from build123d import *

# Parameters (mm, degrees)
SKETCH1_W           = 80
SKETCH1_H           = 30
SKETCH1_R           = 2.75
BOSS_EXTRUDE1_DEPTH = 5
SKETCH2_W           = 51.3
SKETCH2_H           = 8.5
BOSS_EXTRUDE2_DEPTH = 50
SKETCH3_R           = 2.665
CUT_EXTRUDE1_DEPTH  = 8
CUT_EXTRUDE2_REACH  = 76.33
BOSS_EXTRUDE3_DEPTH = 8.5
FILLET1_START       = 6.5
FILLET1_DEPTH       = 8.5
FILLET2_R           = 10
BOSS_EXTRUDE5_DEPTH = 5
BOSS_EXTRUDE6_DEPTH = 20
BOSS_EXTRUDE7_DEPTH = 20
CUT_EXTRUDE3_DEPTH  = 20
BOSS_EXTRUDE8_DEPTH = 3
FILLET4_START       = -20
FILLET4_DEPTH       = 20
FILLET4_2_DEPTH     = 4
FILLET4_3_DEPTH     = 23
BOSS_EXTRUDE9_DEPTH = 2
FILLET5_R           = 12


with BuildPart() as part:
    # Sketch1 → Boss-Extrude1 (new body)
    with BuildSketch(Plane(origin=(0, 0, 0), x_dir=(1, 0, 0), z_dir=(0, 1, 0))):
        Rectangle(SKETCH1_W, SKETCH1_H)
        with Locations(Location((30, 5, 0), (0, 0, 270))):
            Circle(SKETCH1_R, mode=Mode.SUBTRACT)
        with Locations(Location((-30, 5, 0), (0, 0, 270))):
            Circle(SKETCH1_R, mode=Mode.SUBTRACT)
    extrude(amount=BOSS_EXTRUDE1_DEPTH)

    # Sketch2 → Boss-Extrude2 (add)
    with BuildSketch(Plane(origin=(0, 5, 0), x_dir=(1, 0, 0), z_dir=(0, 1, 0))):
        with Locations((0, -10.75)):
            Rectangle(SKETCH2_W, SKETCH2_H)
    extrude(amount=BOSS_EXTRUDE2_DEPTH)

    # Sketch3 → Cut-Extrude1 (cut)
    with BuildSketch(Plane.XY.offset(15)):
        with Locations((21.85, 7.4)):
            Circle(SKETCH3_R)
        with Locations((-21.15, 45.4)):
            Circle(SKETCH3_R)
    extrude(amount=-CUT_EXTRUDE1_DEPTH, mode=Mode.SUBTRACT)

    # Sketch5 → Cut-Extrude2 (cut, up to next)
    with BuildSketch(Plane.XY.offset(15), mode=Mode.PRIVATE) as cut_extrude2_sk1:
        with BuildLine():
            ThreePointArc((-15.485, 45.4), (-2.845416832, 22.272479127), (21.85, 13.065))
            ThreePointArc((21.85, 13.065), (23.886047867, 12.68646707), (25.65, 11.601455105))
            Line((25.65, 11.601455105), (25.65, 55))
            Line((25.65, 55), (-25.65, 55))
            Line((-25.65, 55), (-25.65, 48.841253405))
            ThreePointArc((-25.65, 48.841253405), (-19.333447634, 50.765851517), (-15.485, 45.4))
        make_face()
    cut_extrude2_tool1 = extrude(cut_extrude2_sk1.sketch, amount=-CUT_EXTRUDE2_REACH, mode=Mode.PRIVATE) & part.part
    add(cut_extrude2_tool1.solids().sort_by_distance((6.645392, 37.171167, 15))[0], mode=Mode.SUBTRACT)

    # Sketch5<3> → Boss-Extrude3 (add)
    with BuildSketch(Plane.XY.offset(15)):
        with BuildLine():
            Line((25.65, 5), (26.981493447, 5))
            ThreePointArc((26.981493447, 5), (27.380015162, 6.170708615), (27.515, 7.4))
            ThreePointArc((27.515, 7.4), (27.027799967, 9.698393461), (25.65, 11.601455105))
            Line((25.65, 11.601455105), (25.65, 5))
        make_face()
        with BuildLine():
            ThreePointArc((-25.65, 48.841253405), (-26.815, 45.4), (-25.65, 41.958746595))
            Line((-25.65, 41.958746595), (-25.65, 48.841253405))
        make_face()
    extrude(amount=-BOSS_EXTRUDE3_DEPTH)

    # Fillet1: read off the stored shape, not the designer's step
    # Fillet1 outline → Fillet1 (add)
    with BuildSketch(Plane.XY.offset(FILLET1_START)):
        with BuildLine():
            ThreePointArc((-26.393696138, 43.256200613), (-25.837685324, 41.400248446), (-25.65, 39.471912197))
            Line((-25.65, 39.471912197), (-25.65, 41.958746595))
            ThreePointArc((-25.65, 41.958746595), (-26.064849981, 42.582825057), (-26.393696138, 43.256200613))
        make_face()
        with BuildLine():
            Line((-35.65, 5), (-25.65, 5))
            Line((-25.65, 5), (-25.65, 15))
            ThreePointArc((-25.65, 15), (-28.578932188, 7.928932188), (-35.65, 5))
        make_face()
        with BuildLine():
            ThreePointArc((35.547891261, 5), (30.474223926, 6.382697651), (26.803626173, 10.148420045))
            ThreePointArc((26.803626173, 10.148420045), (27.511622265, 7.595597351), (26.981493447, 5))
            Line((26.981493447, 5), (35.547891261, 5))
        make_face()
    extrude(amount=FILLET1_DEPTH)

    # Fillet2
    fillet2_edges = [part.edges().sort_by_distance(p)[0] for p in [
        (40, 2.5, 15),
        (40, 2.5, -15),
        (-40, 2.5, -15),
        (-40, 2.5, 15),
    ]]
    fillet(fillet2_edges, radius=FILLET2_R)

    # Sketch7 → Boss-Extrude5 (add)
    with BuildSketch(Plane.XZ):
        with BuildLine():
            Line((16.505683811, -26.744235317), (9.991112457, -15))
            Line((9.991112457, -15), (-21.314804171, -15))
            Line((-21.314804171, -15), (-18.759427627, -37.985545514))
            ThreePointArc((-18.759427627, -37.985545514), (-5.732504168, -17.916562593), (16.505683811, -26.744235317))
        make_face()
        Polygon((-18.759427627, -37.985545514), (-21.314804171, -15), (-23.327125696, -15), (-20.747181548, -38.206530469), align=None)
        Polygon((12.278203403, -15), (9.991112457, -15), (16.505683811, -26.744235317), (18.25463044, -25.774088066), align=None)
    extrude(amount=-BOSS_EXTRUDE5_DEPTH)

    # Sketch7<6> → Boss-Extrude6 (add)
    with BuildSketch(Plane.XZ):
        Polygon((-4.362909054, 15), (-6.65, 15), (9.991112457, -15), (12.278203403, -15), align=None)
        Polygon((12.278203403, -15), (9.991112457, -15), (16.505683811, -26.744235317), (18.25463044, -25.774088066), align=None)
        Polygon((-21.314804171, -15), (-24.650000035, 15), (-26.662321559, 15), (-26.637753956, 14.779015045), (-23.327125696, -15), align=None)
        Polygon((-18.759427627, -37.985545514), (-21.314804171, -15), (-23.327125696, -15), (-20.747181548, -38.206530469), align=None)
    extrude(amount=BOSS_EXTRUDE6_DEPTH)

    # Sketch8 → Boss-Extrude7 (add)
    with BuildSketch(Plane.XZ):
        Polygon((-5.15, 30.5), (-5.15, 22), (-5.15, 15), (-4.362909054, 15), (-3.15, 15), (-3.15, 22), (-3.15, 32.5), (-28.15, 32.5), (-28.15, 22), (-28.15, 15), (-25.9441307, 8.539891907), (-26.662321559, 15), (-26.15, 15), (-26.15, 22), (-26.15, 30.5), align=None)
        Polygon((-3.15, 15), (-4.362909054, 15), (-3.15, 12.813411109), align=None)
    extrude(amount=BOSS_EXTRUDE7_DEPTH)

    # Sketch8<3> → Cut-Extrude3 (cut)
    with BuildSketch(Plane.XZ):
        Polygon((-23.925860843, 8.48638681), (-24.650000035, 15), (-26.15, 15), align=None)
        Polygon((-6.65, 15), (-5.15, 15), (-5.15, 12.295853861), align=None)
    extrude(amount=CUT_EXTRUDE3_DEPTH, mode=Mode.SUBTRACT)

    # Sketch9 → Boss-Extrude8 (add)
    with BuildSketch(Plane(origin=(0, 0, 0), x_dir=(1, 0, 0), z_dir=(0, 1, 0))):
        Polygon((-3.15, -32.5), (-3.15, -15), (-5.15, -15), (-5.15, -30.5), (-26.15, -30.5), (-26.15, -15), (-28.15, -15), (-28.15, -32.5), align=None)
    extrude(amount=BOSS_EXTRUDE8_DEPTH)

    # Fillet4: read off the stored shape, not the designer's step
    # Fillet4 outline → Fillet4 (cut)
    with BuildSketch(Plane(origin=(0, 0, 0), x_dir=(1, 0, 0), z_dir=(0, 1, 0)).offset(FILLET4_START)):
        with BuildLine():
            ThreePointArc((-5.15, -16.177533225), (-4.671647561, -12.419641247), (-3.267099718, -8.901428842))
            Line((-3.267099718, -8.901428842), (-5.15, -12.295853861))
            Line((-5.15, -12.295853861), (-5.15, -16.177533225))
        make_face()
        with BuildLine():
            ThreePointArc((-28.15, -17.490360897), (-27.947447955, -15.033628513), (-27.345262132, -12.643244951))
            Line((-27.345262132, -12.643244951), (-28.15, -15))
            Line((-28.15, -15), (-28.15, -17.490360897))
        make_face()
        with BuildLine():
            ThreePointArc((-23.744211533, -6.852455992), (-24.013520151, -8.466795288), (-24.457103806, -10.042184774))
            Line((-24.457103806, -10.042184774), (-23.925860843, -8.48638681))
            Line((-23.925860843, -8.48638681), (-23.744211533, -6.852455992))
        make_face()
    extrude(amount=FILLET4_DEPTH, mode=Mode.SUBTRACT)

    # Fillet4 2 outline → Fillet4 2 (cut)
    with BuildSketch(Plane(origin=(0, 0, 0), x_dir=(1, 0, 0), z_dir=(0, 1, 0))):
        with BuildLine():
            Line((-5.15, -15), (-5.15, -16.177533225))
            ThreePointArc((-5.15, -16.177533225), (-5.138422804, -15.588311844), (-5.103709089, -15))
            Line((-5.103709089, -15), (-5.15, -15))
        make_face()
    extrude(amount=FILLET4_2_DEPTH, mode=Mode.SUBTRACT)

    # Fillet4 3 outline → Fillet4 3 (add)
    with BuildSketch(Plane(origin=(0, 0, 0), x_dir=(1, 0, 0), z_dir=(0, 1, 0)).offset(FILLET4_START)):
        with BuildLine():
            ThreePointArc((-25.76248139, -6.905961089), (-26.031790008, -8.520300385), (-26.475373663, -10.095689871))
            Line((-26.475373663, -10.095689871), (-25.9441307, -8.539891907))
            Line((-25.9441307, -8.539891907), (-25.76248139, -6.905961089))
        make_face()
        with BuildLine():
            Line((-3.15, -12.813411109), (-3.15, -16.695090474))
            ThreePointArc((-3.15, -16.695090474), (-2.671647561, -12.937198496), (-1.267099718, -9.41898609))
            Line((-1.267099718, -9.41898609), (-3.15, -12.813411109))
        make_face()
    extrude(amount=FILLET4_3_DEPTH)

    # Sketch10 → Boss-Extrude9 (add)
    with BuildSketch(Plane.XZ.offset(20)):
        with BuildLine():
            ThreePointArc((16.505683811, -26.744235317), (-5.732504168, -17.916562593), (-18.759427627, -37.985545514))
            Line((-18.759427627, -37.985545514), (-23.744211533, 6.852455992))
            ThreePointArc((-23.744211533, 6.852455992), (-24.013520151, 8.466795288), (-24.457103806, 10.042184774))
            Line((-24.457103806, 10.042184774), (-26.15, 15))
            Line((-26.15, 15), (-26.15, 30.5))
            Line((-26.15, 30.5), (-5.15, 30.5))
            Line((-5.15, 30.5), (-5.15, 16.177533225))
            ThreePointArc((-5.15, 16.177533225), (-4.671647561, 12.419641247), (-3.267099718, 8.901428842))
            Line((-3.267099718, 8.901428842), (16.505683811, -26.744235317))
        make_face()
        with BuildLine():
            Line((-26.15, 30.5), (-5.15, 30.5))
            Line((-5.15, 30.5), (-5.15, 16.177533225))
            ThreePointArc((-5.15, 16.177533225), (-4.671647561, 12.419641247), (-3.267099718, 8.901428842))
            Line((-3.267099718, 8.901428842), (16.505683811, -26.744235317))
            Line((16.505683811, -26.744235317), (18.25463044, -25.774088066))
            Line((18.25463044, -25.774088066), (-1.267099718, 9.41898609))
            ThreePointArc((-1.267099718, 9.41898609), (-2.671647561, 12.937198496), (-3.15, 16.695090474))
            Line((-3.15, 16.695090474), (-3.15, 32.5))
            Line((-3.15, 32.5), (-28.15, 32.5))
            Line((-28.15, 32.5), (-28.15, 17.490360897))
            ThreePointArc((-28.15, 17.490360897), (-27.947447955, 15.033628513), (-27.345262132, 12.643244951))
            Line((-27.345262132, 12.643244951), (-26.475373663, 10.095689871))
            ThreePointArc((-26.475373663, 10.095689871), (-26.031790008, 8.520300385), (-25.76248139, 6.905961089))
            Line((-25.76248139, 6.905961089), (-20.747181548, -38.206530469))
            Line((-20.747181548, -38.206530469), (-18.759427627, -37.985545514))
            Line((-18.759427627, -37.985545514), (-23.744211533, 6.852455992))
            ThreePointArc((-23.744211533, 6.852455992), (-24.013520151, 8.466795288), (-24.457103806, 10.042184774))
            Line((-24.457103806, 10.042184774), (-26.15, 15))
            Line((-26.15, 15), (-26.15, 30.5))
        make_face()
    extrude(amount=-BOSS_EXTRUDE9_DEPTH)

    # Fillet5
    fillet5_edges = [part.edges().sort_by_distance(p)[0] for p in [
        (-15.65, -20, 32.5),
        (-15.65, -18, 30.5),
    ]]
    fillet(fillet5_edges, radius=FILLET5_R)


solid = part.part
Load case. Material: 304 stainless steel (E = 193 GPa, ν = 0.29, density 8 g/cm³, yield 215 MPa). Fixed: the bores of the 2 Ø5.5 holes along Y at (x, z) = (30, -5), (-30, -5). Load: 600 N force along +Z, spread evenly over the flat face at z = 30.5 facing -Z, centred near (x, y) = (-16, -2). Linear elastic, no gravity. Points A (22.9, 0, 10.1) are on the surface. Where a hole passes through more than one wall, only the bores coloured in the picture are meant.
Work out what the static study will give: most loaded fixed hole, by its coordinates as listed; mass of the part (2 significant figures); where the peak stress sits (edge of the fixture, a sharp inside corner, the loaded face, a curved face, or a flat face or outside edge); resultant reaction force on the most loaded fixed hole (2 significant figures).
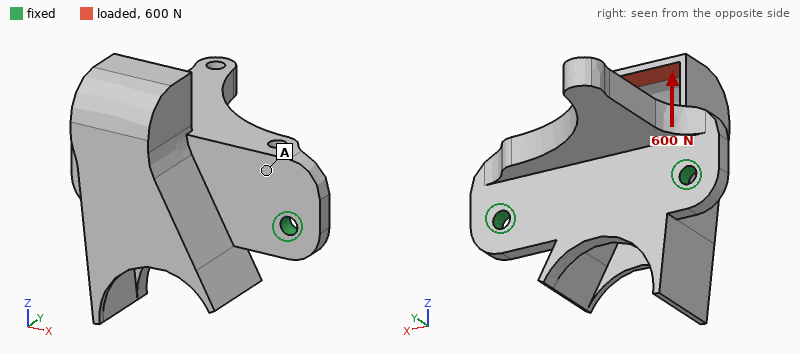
(-30, -5)
250 g
the loaded face
460 N
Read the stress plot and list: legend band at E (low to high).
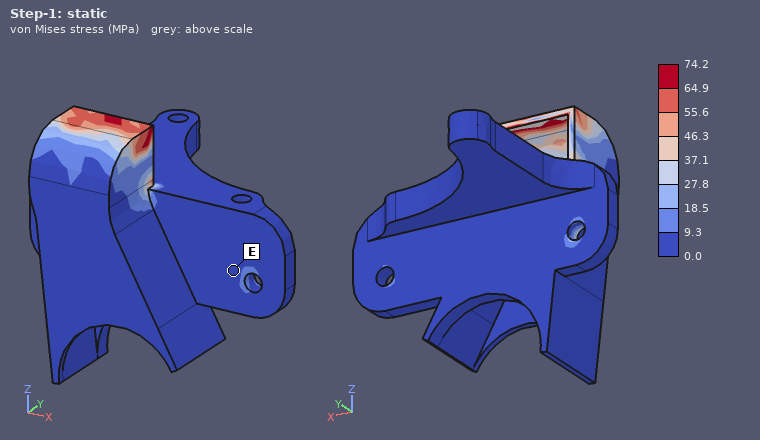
0.0 to 9.3 MPa
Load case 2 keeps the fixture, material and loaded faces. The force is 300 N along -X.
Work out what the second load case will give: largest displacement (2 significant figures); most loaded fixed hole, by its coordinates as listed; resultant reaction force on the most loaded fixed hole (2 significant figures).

29 µm
(30, -5)
270 N
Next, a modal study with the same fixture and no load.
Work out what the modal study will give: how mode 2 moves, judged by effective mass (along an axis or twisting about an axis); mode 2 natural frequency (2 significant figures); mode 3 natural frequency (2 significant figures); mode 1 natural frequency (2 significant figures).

along X
3300 Hz
4500 Hz
2000 Hz
